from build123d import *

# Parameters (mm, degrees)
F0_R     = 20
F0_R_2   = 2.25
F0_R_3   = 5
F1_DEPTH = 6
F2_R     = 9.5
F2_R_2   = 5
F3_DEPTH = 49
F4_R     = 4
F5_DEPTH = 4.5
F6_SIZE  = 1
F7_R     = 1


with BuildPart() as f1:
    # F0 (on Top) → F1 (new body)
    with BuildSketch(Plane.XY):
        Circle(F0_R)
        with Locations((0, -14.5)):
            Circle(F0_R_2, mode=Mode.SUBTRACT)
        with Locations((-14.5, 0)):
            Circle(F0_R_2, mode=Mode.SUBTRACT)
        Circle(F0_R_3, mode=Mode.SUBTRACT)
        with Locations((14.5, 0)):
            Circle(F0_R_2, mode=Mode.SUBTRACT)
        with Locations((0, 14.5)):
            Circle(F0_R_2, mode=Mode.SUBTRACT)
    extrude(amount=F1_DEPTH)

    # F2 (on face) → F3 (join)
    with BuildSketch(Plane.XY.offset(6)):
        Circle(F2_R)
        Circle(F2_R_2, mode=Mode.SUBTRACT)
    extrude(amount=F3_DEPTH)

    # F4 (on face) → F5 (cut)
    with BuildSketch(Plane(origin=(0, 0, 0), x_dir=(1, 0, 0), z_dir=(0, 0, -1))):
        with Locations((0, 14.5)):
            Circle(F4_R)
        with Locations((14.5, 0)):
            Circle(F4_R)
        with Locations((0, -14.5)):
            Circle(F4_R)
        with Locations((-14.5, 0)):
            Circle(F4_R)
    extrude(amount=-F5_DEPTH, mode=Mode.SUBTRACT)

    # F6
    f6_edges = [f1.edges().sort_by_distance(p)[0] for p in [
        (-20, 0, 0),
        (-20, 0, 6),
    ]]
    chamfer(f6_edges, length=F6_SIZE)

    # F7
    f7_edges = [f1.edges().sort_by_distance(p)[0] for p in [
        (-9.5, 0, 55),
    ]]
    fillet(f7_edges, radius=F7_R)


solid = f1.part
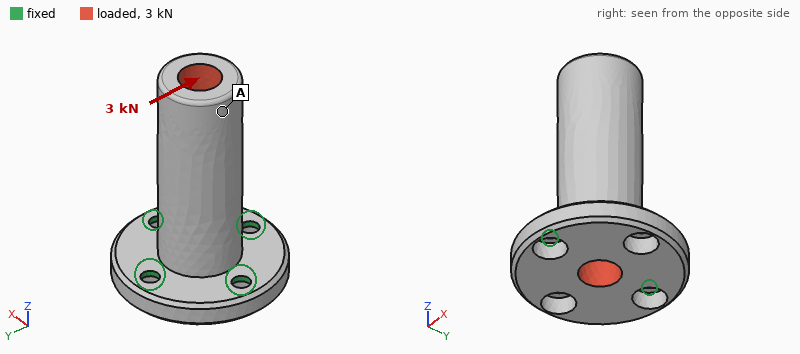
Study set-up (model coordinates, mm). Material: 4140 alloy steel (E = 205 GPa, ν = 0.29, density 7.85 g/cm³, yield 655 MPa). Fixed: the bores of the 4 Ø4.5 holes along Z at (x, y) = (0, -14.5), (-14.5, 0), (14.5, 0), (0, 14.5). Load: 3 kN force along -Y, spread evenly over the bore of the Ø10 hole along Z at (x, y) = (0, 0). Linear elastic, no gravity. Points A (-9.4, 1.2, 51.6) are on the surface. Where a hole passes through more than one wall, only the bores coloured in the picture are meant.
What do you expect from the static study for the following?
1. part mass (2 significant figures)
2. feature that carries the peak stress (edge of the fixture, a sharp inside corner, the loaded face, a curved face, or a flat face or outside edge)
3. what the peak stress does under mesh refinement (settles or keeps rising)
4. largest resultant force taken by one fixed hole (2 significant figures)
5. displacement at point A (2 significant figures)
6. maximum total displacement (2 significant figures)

130 g
edge of the fixture
keeps rising
2.4 kN
79 µm
87 µm
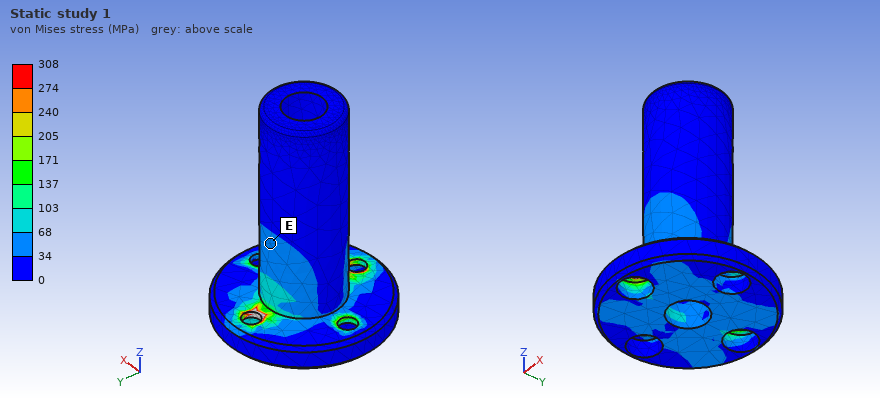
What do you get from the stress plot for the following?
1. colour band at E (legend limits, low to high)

34 to 68 MPa
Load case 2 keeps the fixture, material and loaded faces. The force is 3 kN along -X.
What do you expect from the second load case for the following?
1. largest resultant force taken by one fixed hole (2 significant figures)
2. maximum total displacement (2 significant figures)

2.4 kN
87 µm
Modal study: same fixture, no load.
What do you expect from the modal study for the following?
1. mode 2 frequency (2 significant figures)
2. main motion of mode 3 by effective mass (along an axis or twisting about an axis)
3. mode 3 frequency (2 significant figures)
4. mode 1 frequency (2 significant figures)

3800 Hz
along Z
14 kHz
3800 Hz
